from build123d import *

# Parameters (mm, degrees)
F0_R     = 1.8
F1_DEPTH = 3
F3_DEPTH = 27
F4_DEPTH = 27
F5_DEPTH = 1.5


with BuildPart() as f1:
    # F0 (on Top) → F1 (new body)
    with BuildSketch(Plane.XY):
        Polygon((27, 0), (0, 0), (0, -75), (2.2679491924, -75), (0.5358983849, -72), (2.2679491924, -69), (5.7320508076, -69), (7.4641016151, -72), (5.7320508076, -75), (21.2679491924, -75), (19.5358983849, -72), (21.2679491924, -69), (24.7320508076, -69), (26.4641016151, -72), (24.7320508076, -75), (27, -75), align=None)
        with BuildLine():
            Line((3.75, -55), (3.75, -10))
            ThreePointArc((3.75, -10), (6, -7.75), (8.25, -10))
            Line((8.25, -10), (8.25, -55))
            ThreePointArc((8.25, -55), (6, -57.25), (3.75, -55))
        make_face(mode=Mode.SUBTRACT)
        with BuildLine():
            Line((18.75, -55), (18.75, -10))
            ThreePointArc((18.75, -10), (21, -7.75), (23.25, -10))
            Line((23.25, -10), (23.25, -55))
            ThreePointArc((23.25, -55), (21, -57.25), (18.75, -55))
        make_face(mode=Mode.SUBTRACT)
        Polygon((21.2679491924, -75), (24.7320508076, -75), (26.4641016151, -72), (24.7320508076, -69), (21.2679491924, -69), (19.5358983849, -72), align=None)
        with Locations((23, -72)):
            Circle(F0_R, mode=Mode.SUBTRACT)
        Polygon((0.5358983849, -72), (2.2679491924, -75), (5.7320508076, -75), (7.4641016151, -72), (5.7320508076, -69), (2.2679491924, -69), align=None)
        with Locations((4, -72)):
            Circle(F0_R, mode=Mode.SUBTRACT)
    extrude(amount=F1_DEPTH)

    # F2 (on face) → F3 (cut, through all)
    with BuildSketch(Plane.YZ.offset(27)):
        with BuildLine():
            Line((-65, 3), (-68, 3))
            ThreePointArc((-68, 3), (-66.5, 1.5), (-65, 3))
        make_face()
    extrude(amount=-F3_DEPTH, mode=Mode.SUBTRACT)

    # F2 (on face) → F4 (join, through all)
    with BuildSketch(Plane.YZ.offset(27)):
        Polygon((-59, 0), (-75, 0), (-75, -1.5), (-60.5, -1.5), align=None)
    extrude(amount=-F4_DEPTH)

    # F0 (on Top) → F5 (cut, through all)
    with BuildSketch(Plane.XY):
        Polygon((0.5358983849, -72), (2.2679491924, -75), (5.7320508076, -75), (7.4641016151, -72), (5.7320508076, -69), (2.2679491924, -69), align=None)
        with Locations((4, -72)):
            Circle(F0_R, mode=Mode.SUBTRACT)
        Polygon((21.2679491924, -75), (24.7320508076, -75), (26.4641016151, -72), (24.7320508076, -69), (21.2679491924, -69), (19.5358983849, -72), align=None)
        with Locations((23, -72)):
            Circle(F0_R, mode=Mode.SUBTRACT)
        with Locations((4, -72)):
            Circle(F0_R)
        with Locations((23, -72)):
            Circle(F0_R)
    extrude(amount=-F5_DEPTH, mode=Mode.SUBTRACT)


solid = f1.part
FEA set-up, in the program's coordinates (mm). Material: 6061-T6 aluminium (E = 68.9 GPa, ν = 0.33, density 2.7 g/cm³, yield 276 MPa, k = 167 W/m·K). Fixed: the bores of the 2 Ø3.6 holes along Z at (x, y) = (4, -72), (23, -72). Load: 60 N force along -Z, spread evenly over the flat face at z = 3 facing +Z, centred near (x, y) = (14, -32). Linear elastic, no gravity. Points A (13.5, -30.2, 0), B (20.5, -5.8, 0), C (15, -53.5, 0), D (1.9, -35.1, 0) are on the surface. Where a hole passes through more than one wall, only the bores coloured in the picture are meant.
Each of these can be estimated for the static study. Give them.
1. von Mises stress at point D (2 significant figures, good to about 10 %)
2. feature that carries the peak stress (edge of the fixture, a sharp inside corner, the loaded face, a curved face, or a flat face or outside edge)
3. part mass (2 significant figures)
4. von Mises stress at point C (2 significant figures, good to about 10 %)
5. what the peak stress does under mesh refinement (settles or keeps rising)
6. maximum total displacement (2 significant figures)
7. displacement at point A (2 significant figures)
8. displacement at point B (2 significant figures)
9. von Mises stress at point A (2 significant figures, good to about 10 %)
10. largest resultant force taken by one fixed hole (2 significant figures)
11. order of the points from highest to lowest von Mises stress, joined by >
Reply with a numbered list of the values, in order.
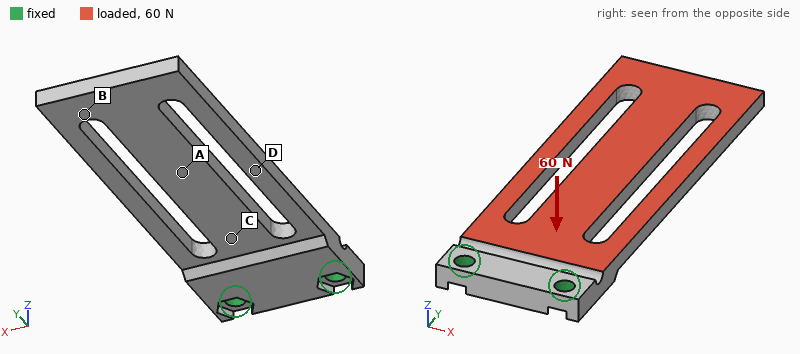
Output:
1. 23 MPa
2. edge of the fixture
3. 14 g
4. 47 MPa
5. keeps rising
6. 0.77 mm
7. 0.32 mm
8. 0.68 mm
9. 17 MPa
10. 34 N
11. C > D > A > B
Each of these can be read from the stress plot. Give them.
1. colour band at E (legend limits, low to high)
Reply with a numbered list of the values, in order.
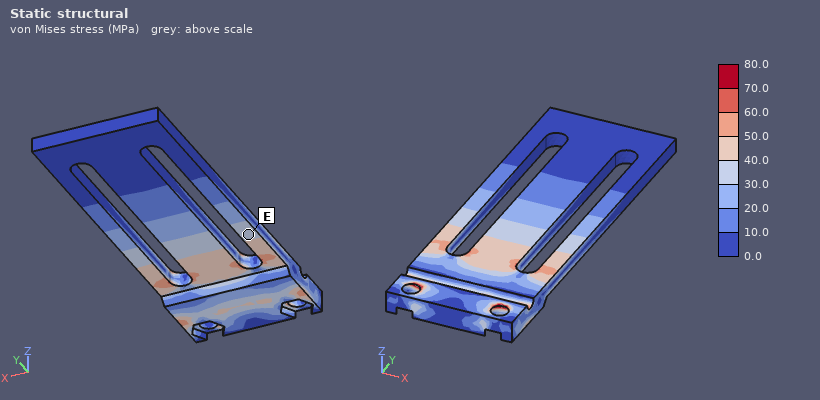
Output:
1. 30.0 to 40.0 MPa
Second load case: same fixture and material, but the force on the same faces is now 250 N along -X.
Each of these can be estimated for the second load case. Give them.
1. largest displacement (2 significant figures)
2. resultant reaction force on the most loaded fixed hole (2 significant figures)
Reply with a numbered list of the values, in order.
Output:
1. 0.13 mm
2. 490 N
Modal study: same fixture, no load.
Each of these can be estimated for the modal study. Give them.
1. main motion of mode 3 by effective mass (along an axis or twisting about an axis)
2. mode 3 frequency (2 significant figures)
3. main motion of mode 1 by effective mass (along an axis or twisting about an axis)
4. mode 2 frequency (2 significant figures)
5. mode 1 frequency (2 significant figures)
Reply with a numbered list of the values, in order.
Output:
1. along X
2. 2500 Hz
3. along Z
4. 2300 Hz
5. 520 Hz
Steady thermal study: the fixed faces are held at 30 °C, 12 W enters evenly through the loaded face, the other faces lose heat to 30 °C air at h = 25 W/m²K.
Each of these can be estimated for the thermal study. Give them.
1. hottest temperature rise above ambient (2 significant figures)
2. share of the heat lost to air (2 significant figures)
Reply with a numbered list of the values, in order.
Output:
1. 38 K
2. 14 %
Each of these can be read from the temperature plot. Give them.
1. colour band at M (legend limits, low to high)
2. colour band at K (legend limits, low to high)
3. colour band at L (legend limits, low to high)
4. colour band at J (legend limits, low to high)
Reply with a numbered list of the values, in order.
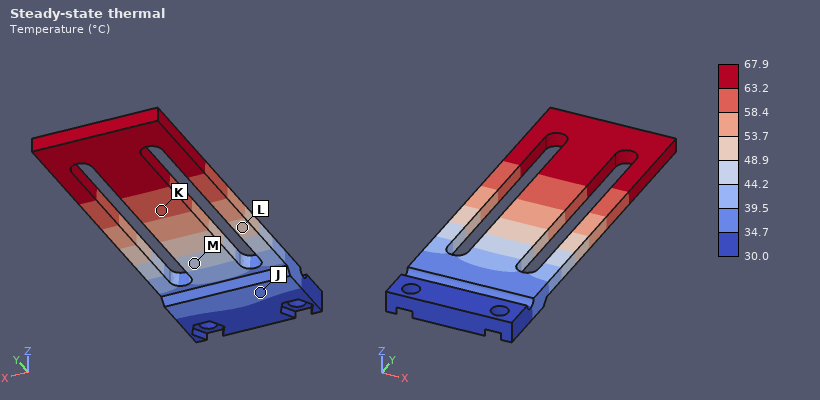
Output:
1. 44.2 to 48.9 °C
2. 58.4 to 63.2 °C
3. 48.9 to 53.7 °C
4. 34.7 to 39.5 °C
